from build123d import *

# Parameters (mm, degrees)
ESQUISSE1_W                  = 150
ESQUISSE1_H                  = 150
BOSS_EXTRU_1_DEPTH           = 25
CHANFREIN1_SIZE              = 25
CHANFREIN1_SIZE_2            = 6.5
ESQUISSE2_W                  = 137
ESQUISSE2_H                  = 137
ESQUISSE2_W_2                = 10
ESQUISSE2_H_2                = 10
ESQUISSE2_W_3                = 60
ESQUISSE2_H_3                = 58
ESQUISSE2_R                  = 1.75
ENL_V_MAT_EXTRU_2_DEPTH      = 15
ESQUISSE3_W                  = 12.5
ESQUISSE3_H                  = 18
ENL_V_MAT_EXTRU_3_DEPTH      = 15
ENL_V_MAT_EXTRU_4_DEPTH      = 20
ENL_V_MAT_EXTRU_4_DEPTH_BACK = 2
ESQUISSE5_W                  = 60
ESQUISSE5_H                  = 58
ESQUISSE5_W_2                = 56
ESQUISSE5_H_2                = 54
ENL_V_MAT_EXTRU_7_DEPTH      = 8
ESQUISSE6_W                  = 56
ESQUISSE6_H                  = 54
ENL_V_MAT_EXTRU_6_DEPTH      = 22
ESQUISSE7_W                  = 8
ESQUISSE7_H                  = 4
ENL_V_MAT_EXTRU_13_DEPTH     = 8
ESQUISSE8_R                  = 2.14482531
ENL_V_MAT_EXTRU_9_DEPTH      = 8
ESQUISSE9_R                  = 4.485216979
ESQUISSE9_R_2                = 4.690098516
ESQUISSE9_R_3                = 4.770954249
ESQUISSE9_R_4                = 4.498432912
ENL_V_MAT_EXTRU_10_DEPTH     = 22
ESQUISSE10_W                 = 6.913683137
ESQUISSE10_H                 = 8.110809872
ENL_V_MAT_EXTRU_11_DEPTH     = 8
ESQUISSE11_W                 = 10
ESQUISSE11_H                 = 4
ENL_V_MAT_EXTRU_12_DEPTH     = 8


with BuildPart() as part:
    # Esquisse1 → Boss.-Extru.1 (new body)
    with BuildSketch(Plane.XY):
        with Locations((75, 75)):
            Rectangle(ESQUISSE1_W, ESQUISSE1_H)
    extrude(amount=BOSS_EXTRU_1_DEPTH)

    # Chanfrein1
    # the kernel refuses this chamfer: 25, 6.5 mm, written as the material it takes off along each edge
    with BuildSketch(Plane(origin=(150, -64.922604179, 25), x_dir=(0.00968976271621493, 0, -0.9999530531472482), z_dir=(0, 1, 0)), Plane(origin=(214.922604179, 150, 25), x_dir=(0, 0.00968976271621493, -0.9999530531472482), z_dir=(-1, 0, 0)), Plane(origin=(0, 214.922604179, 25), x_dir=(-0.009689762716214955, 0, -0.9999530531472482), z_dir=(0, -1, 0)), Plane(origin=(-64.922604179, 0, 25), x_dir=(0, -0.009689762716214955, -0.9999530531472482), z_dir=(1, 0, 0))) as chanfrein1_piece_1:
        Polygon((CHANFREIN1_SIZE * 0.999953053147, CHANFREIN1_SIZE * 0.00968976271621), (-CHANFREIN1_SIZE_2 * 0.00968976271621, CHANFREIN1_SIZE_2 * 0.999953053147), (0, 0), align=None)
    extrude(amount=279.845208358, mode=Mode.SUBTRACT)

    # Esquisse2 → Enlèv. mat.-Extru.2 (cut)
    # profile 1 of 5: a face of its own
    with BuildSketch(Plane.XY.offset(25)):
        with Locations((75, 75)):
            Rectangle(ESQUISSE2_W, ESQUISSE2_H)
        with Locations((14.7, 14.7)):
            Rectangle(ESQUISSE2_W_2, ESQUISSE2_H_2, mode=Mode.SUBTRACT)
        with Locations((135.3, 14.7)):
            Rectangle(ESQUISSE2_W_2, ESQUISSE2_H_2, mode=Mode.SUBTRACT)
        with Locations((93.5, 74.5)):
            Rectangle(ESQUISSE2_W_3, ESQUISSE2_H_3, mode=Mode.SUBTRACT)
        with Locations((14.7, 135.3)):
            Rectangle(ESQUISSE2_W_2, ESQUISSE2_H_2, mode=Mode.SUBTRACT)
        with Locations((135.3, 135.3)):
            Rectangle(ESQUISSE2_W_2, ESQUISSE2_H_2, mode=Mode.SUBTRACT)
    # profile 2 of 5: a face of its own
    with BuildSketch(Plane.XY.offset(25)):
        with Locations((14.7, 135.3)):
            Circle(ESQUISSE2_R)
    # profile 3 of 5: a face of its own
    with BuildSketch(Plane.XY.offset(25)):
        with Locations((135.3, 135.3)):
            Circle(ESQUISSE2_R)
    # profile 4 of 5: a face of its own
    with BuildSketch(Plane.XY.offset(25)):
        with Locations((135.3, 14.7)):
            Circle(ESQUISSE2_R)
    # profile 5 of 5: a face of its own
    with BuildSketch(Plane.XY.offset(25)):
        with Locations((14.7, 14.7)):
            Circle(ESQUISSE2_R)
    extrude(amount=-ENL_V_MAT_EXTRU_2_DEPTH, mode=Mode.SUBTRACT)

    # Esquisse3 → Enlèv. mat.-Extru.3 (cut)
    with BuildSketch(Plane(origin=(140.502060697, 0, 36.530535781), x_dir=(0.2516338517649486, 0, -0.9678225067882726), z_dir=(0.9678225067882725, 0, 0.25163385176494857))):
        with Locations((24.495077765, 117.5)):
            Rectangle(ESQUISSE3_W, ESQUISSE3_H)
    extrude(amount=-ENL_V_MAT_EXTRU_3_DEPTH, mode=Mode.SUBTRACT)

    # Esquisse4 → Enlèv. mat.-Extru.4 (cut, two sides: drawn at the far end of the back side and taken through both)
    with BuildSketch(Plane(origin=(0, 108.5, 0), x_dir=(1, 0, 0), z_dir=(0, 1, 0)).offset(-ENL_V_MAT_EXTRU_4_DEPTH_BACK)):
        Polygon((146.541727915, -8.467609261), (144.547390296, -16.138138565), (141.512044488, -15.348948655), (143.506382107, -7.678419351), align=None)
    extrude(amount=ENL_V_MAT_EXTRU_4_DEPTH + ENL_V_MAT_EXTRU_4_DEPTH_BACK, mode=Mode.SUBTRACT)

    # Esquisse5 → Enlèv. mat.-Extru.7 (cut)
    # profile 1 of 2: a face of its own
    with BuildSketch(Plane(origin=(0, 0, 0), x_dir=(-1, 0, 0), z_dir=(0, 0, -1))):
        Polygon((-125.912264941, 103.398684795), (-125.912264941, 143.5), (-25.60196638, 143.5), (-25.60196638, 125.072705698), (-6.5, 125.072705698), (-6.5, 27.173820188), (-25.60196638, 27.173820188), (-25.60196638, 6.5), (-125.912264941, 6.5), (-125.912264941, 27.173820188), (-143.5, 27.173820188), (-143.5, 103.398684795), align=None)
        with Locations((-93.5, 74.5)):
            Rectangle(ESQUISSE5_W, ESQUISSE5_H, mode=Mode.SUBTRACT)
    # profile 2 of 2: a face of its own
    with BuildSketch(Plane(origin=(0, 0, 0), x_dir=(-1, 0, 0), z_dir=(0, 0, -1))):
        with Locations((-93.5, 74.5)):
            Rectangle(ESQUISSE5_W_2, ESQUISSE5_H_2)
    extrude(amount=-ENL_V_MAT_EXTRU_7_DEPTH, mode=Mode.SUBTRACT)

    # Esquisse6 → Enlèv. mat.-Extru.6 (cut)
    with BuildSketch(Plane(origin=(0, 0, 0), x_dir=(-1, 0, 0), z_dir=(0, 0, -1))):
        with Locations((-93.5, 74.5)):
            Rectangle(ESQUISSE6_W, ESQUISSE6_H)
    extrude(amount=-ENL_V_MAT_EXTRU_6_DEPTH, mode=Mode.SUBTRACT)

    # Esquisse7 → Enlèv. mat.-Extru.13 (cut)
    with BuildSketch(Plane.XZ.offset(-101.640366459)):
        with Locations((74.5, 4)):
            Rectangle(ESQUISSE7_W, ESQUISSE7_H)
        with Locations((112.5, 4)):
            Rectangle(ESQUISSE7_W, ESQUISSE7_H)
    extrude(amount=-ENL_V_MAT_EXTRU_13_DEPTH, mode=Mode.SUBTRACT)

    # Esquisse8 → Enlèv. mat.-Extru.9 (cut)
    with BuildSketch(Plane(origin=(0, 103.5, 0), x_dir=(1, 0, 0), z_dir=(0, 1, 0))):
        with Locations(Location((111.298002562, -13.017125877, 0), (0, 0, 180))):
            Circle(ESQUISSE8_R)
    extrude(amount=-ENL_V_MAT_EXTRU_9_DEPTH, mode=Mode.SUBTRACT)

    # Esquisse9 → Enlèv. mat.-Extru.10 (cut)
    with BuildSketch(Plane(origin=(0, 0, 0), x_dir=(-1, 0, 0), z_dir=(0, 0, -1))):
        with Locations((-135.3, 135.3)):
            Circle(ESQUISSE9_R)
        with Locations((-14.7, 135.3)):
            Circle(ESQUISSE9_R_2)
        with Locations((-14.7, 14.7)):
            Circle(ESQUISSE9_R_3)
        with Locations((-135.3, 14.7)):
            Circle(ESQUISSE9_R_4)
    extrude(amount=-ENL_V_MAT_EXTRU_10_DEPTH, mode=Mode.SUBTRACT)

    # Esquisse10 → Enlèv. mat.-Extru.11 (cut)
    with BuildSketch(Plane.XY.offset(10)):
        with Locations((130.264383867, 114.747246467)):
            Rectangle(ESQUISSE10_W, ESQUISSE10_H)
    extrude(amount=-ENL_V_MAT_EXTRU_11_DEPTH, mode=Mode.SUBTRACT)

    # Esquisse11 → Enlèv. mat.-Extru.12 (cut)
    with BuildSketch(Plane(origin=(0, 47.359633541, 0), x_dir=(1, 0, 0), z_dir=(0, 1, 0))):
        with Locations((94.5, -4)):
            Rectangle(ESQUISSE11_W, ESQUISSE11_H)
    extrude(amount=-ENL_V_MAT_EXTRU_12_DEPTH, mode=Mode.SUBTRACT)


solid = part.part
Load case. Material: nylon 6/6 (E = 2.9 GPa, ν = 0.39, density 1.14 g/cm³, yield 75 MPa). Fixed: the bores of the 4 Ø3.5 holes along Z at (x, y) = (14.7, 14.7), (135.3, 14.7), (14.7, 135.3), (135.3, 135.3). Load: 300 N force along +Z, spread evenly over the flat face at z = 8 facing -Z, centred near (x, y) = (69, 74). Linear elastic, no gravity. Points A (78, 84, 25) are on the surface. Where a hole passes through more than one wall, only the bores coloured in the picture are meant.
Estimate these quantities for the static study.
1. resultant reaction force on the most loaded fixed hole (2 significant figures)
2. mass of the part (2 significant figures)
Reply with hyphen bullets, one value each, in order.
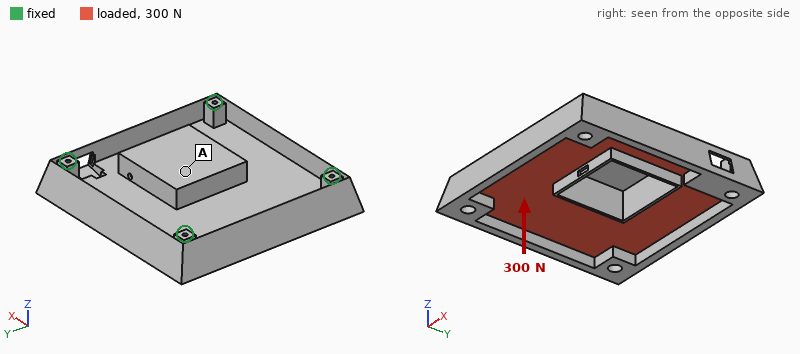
- 96 N
- 120 g
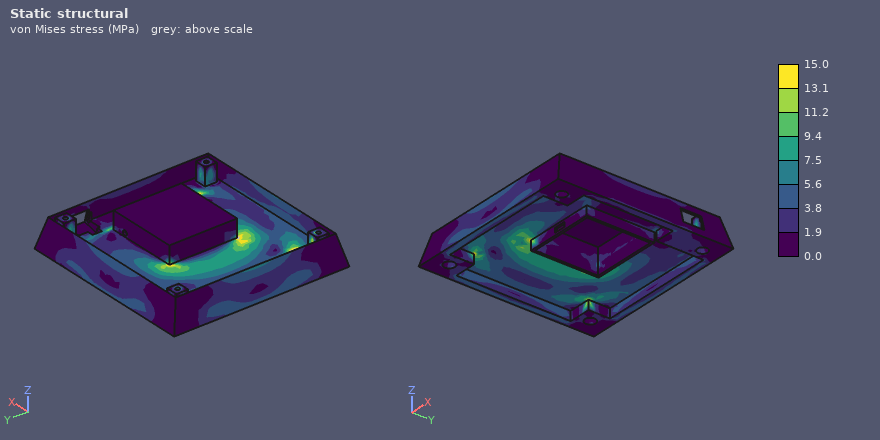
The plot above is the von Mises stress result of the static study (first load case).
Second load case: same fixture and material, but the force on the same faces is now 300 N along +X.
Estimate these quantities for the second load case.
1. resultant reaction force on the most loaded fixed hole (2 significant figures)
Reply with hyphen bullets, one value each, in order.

- 82 N
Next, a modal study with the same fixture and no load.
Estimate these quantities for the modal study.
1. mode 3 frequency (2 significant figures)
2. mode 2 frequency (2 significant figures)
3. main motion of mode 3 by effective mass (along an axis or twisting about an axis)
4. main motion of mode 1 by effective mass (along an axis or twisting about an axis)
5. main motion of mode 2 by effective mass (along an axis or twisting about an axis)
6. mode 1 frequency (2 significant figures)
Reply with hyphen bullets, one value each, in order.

- 610 Hz
- 560 Hz
- along X
- along Z
- along Y
- 290 Hz
